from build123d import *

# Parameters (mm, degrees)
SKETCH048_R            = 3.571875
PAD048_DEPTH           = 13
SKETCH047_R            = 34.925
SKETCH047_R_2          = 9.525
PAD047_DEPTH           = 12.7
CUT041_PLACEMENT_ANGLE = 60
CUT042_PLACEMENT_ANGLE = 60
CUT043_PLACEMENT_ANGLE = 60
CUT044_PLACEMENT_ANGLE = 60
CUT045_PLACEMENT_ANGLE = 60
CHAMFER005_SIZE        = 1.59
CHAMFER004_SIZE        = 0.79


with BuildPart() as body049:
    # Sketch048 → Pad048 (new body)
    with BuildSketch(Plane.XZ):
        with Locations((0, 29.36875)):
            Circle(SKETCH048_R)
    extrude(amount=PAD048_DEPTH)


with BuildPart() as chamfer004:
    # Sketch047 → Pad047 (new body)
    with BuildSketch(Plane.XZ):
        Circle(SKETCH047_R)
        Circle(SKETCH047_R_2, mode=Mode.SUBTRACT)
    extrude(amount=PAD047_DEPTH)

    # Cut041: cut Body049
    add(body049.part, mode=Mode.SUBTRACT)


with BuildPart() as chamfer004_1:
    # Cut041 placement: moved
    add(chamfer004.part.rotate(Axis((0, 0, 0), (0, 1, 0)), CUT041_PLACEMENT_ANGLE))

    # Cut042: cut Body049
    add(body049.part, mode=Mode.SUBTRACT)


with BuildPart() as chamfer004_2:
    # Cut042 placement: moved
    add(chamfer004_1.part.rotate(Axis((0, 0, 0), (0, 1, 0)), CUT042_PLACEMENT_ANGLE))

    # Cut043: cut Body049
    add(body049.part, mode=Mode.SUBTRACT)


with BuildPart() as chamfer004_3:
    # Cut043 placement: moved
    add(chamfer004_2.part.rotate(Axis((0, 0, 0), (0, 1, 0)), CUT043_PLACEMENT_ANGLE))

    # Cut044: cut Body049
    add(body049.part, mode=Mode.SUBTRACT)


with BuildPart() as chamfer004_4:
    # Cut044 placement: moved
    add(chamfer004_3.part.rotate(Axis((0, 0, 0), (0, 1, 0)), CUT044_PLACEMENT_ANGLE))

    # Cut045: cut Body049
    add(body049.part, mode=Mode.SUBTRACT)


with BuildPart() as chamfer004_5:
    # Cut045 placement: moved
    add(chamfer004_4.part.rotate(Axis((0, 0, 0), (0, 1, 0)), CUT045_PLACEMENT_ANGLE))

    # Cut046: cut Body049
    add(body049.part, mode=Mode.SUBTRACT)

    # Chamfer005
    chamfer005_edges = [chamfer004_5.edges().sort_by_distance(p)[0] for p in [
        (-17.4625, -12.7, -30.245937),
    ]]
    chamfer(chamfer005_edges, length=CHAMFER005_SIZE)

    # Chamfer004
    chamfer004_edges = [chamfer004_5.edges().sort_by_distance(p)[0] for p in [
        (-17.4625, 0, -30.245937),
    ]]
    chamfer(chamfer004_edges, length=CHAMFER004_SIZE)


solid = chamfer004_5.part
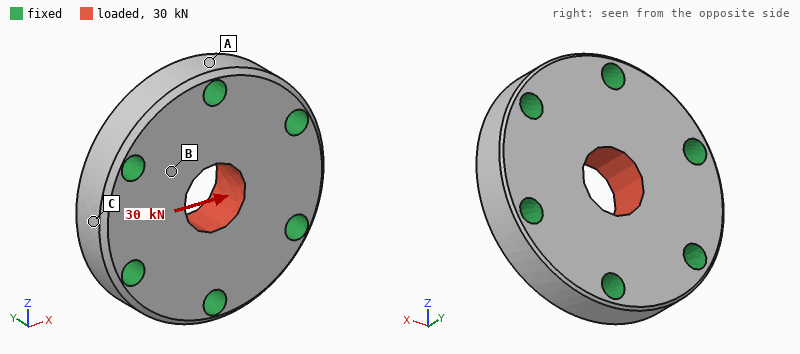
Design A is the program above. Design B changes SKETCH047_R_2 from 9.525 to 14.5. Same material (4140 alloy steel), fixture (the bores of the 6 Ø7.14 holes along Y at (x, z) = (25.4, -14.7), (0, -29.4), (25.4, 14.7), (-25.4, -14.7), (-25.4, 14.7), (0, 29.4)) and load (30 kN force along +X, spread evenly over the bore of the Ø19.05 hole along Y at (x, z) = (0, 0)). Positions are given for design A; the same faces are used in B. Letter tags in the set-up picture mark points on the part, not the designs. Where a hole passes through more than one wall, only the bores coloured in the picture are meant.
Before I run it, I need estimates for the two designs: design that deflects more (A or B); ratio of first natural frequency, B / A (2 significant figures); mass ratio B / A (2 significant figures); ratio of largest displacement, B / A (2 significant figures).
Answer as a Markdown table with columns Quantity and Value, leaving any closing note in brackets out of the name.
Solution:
| Quantity | Value |
|---|---|
| design that deflects more | A |
| ratio of first natural frequency, B / A | 1.3 |
| mass ratio B / A | 0.89 |
| ratio of largest displacement, B / A | 0.70 |
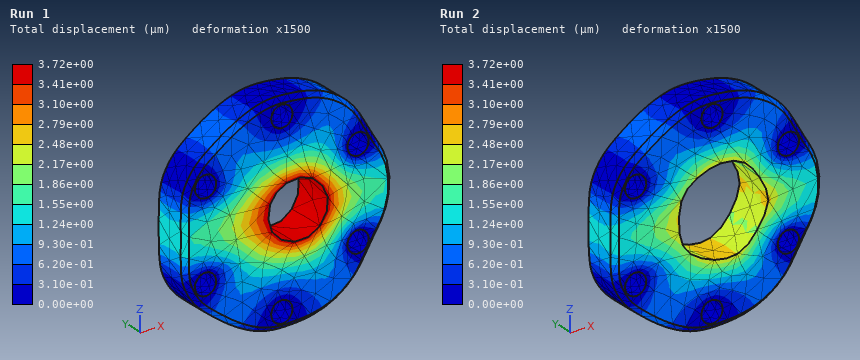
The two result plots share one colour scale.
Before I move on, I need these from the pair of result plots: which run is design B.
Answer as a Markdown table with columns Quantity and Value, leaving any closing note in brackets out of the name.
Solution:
| Quantity | Value |
|---|---|
| which run is design B | Run 2 |
